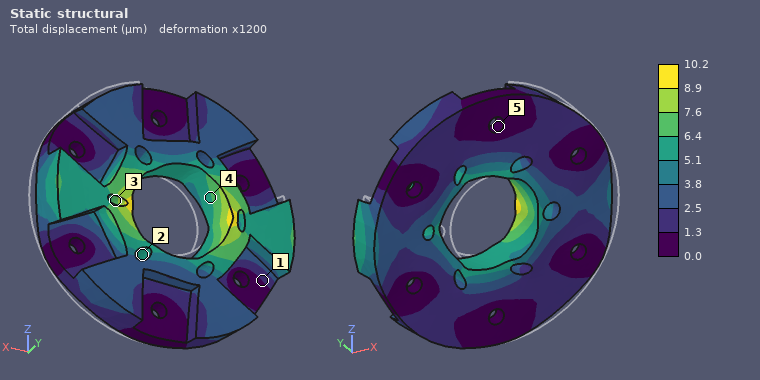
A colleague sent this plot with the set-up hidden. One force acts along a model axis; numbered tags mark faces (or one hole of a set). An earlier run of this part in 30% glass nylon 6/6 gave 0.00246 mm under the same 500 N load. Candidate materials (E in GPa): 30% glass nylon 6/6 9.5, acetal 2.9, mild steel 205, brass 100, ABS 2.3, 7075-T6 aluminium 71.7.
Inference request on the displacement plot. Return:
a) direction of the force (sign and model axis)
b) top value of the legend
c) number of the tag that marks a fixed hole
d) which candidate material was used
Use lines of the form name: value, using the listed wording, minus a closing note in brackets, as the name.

direction of the force: -X
top value of the legend: 10.2 µm
number of the tag that marks a fixed hole: 5
which candidate material was used: ABS
